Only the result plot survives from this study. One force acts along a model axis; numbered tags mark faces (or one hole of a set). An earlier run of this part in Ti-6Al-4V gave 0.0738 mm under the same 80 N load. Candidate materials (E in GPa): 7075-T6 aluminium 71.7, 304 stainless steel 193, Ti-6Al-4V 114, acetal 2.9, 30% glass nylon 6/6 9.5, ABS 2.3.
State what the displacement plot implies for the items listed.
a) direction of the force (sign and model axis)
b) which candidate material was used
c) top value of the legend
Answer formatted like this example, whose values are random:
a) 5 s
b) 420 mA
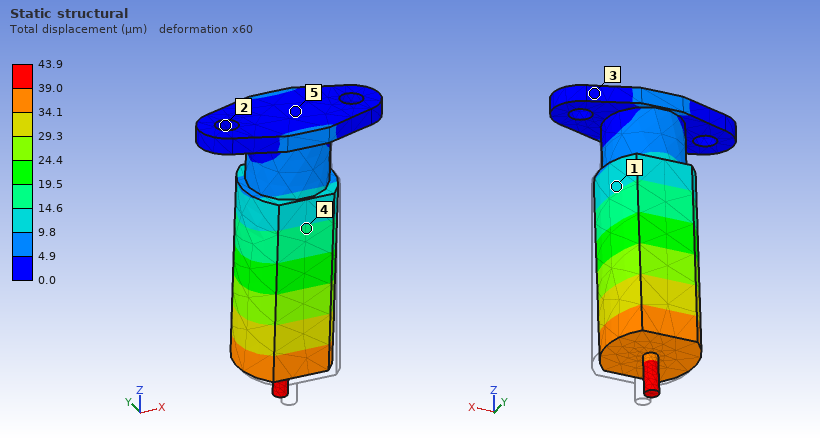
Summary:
a) +Y
b) 304 stainless steel
c) 43.9 µm
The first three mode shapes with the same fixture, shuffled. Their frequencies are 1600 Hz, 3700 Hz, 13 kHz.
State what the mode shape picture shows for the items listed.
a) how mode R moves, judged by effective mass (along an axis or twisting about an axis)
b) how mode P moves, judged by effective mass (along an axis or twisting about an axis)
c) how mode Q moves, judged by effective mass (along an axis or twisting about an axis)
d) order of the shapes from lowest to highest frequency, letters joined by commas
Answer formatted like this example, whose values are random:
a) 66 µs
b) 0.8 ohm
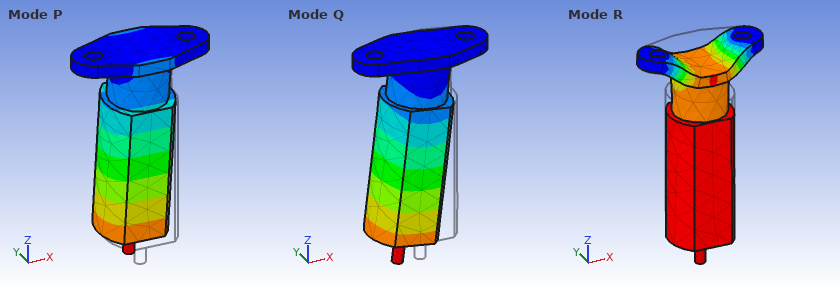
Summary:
a) along Z
b) along Y
c) along X
d) P, Q, R
